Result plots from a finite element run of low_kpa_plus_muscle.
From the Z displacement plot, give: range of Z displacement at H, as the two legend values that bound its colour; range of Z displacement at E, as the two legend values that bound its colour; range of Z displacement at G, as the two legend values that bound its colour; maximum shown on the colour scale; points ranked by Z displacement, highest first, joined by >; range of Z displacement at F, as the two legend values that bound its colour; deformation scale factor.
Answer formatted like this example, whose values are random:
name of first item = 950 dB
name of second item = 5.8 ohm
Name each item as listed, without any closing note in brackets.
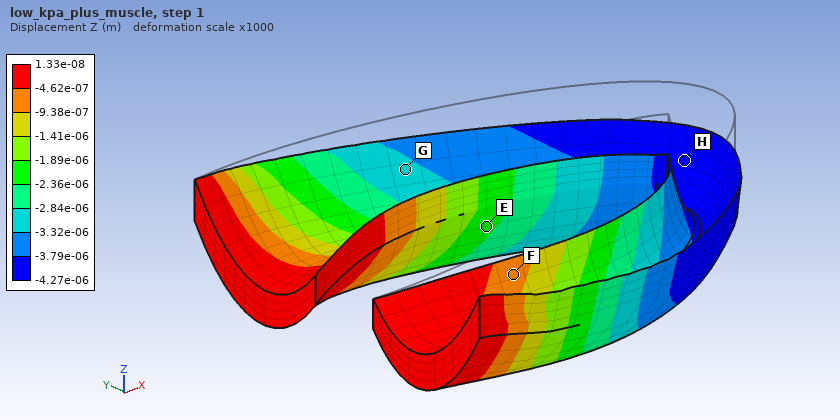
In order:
range of Z displacement at H, as the two legend values that bound its colour = -4.27e-06 to -3.79e-06 m
range of Z displacement at E, as the two legend values that bound its colour = -2.36e-06 to -1.89e-06 m
range of Z displacement at G, as the two legend values that bound its colour = -3.32e-06 to -2.84e-06 m
maximum shown on the colour scale = 1.33e-08 m
points ranked by Z displacement, highest first, joined by > = F > E > G > H
range of Z displacement at F, as the two legend values that bound its colour = -9.38e-07 to -4.62e-07 m
deformation scale factor = 1000
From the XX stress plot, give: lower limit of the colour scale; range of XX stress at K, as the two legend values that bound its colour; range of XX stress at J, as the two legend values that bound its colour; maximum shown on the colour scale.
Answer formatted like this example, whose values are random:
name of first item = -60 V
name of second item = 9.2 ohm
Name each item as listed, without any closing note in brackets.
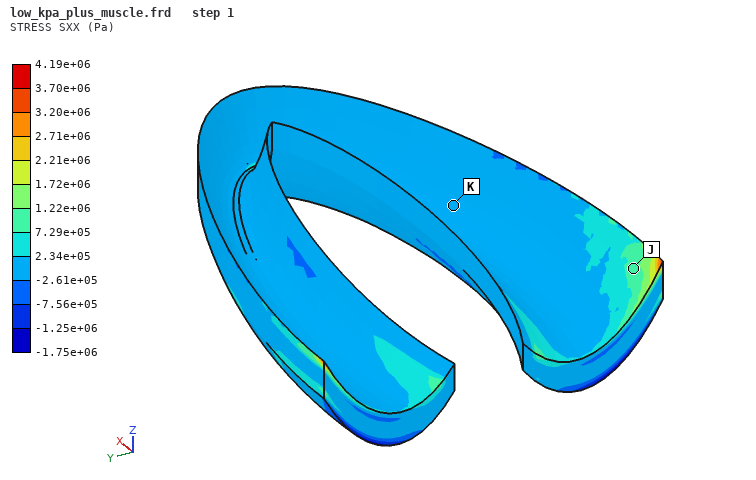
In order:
lower limit of the colour scale = -1.75e+06 Pa
range of XX stress at K, as the two legend values that bound its colour = -2.61e+05 to 2.34e+05 Pa
range of XX stress at J, as the two legend values that bound its colour = 7.29e+05 to 1.22e+06 Pa
maximum shown on the colour scale = 4.19e+06 Pa
